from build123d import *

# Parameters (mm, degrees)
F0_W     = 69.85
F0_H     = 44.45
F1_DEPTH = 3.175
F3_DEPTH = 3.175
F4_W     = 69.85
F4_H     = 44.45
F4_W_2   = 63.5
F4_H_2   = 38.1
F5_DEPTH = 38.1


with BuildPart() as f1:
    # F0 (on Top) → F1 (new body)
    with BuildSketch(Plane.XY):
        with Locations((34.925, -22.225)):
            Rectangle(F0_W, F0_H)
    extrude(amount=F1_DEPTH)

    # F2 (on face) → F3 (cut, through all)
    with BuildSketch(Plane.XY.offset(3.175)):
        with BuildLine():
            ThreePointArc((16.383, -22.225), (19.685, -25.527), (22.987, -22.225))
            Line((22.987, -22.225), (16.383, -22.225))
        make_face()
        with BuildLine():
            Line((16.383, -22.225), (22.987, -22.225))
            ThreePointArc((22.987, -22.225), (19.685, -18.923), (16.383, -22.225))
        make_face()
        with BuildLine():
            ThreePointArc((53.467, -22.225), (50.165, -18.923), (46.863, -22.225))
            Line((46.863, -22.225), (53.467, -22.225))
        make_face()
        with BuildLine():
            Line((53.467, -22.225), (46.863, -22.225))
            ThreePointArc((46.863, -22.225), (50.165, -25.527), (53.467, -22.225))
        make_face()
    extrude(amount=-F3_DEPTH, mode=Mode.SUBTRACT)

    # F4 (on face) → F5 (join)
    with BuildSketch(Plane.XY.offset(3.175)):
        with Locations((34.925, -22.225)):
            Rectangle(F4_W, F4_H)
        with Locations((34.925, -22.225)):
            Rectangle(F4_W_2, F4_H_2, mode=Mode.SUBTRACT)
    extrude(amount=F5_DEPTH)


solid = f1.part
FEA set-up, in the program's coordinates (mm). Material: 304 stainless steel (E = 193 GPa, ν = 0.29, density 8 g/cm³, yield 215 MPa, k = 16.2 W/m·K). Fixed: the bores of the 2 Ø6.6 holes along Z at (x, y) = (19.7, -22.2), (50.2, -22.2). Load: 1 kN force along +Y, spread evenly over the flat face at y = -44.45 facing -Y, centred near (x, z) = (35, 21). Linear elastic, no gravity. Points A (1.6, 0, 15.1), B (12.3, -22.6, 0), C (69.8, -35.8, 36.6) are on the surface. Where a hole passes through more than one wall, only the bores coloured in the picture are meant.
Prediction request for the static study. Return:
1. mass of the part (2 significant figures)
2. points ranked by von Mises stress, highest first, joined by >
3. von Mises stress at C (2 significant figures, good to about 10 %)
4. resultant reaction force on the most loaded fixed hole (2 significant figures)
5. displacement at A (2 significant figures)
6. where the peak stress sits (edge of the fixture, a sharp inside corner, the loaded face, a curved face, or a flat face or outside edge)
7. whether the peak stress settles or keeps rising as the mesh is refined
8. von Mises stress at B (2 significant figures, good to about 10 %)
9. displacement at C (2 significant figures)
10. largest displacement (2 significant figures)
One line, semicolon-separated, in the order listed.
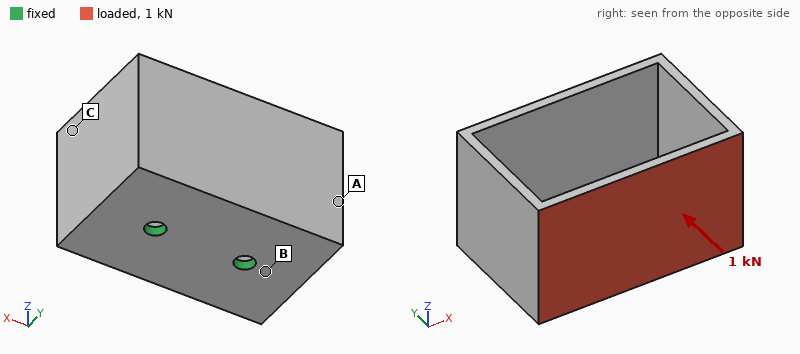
290 g; B > C > A; 26 MPa; 510 N; 0.048 mm; edge of the fixture; keeps rising; 49 MPa; 0.073 mm; 0.14 mm
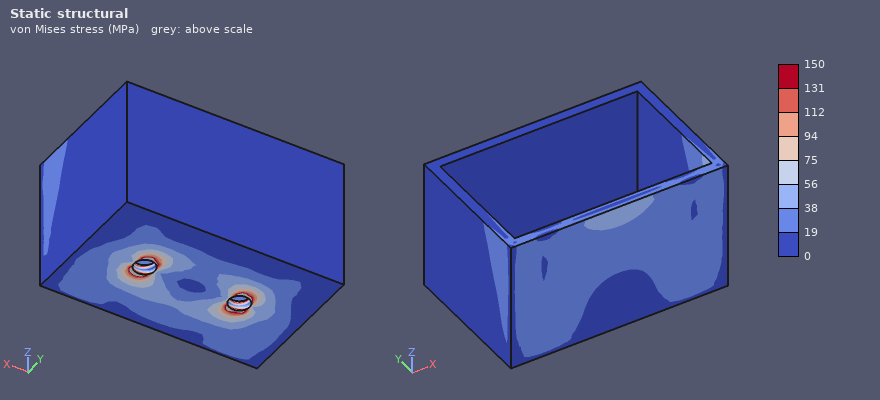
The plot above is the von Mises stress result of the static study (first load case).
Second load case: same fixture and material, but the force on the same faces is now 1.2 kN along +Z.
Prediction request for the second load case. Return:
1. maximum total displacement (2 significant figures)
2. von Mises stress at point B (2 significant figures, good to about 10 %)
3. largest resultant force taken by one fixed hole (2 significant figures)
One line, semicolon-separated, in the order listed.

0.13 mm; 82 MPa; 610 N
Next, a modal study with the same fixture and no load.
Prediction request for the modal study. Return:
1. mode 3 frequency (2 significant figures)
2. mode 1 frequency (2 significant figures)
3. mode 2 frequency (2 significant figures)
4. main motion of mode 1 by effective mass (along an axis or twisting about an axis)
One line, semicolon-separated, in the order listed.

2000 Hz; 1100 Hz; 1900 Hz; along Y
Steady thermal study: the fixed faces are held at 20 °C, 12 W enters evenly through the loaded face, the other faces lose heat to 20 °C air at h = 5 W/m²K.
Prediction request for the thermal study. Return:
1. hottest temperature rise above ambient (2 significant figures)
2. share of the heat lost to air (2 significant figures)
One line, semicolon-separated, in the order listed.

79 K; 26 %
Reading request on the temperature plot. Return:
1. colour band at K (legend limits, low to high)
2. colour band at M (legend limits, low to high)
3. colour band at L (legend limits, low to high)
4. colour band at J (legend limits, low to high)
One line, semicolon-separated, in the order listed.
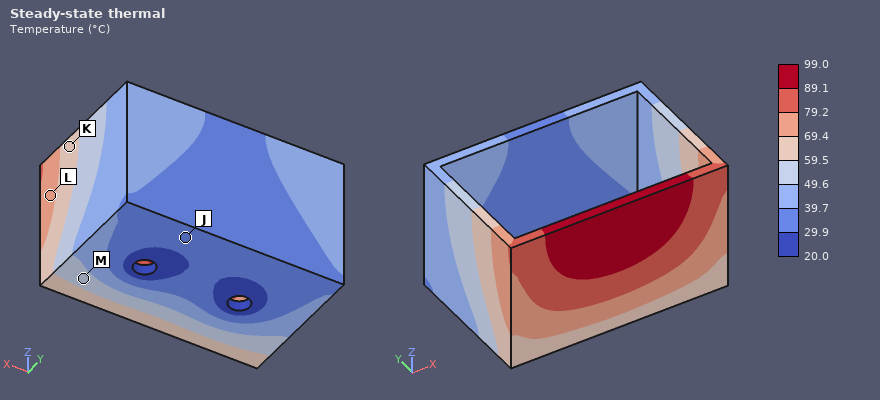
59.5 to 69.4 °C; 49.6 to 59.5 °C; 69.4 to 79.2 °C; 29.9 to 39.7 °C
